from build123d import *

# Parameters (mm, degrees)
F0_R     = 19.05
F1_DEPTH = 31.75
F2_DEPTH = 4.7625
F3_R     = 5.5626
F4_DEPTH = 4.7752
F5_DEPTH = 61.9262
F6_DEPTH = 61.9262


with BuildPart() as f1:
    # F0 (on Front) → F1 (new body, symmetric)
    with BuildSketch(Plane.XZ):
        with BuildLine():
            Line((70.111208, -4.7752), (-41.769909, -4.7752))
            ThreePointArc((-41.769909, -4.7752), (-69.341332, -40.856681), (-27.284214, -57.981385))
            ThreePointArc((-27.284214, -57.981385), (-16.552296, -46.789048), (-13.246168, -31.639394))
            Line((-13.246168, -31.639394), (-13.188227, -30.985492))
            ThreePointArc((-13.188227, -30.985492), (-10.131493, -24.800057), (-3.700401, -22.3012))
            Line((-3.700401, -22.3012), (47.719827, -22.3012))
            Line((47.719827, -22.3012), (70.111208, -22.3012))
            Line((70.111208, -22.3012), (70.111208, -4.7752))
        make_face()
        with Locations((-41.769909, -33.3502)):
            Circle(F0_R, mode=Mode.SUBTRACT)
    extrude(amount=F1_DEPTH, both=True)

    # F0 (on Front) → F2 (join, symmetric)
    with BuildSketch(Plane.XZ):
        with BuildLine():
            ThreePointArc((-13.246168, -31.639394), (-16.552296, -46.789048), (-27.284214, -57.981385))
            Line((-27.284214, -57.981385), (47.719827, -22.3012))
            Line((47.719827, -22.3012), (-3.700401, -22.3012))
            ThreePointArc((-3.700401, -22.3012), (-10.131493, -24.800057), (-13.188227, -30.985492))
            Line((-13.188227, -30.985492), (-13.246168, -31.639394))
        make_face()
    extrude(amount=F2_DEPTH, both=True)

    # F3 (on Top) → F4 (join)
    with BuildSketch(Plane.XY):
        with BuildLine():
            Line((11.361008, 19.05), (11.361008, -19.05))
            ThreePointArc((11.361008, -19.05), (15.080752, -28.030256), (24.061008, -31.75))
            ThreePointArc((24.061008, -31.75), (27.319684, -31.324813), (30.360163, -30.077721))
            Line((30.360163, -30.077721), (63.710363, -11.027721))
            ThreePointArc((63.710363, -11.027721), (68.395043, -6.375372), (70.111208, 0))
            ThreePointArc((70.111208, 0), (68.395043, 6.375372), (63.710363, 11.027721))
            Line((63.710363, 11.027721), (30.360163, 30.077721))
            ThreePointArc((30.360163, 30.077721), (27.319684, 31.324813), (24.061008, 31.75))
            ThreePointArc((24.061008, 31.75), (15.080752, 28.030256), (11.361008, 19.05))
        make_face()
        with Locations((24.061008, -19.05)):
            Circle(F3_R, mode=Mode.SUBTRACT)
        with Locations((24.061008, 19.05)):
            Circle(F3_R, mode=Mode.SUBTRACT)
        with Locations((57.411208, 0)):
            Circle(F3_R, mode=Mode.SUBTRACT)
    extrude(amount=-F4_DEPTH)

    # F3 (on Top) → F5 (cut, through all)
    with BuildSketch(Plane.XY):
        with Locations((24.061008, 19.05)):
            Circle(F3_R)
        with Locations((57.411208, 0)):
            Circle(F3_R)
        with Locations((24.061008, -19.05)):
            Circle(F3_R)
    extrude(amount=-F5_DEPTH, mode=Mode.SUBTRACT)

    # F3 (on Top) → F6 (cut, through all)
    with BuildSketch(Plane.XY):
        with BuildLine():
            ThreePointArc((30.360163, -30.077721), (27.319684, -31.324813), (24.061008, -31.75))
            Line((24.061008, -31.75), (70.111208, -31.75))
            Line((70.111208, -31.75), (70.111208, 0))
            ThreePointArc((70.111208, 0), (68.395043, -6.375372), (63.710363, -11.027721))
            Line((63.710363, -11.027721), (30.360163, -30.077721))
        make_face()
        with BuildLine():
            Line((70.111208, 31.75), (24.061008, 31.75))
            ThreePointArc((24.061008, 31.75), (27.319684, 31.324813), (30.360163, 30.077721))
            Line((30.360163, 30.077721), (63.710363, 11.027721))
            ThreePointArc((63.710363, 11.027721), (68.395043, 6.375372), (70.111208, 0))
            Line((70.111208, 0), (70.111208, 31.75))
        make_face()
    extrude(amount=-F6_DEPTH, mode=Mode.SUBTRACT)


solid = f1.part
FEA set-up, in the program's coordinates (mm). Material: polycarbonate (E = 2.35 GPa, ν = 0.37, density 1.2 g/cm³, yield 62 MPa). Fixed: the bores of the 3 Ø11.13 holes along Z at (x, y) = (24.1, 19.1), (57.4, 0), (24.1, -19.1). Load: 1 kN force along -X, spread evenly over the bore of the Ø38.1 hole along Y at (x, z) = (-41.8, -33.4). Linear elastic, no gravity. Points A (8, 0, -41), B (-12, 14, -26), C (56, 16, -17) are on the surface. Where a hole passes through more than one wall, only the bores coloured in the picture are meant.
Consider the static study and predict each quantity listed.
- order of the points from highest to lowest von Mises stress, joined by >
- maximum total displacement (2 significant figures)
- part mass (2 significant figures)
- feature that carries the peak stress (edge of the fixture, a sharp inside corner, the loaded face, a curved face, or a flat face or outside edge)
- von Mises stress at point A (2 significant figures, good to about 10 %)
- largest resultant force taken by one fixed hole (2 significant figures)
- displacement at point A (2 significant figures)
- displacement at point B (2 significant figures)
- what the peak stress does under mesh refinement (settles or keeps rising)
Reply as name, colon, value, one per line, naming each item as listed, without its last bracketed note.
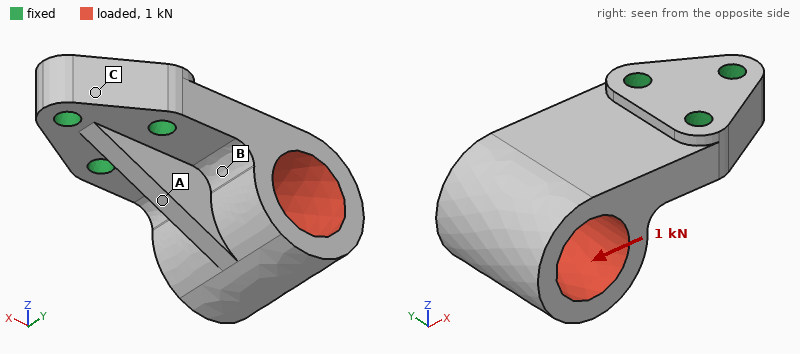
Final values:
order of the points from highest to lowest von Mises stress, joined by >: A > B > C
maximum total displacement: 0.44 mm
part mass: 230 g
feature that carries the peak stress: edge of the fixture
von Mises stress at point A: 4.9 MPa
largest resultant force taken by one fixed hole: 400 N
displacement at point A: 0.11 mm
displacement at point B: 0.11 mm
what the peak stress does under mesh refinement: keeps rising
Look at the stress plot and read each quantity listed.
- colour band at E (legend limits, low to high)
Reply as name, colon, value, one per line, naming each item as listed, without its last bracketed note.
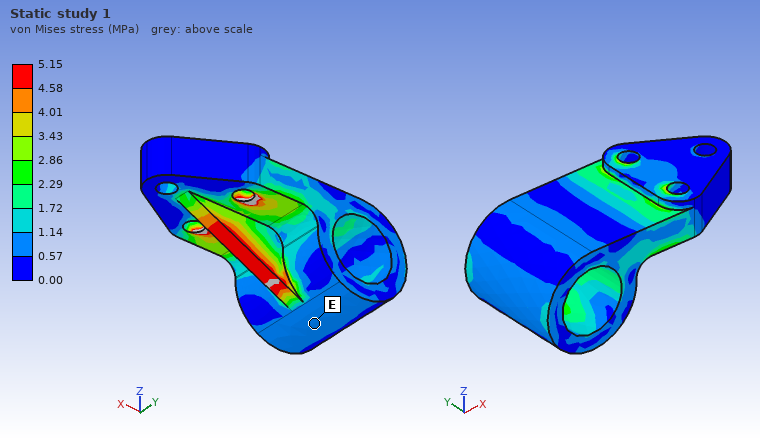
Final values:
colour band at E: 0.57 to 1.14 MPa
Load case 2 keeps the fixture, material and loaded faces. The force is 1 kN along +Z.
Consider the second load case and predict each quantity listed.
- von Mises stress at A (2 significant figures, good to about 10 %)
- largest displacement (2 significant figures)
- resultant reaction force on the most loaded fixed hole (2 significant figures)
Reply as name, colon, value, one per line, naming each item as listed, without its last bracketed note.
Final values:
von Mises stress at A: 9.1 MPa
largest displacement: 1.2 mm
resultant reaction force on the most loaded fixed hole: 750 N
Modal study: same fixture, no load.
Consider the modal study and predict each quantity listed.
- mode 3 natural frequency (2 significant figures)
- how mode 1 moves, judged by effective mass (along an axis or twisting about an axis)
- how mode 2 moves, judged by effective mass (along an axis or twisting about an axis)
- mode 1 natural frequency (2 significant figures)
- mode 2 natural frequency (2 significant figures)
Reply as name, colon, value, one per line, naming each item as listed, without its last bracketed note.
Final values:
mode 3 natural frequency: 1300 Hz
how mode 1 moves, judged by effective mass: along Z
how mode 2 moves, judged by effective mass: along Y
mode 1 natural frequency: 470 Hz
mode 2 natural frequency: 820 Hz
